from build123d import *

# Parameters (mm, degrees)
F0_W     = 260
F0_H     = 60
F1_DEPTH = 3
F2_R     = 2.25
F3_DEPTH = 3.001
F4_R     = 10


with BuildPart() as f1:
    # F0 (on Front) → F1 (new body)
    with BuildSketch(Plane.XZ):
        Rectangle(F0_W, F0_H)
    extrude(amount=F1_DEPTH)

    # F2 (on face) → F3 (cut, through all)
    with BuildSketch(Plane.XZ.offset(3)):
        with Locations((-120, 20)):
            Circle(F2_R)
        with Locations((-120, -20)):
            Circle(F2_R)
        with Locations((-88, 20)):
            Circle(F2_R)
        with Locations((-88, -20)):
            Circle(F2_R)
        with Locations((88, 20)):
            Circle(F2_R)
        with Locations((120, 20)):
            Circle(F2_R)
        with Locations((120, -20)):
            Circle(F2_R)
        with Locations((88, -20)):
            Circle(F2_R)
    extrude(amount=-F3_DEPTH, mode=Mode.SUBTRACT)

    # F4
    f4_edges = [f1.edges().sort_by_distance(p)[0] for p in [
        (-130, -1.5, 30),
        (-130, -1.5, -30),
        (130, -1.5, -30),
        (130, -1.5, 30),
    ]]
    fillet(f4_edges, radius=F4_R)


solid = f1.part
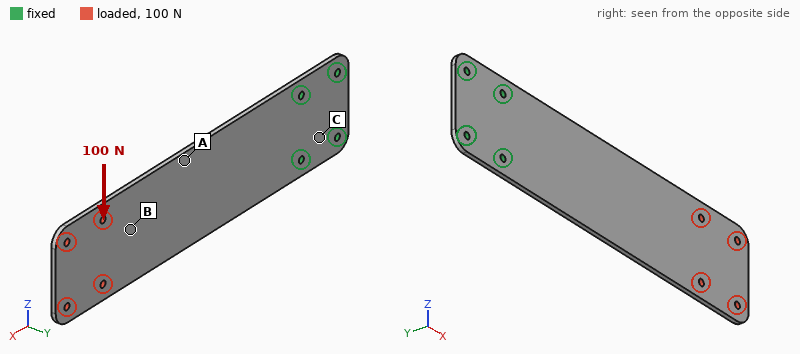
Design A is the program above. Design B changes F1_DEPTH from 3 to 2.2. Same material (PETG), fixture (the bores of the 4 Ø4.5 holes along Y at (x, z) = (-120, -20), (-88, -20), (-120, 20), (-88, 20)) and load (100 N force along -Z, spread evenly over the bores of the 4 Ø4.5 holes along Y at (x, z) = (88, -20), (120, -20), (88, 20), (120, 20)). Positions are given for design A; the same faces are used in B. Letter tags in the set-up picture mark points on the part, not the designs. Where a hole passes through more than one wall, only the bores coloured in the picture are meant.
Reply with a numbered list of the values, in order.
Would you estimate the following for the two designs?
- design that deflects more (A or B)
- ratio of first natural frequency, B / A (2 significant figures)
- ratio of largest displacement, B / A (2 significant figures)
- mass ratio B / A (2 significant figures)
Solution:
1. B
2. 0.74
3. 1.4
4. 0.73
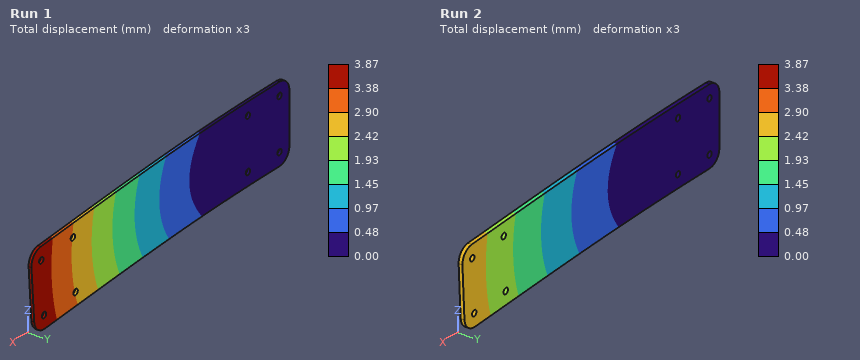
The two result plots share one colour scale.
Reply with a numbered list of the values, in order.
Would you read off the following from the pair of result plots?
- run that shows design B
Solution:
1. Run 1
